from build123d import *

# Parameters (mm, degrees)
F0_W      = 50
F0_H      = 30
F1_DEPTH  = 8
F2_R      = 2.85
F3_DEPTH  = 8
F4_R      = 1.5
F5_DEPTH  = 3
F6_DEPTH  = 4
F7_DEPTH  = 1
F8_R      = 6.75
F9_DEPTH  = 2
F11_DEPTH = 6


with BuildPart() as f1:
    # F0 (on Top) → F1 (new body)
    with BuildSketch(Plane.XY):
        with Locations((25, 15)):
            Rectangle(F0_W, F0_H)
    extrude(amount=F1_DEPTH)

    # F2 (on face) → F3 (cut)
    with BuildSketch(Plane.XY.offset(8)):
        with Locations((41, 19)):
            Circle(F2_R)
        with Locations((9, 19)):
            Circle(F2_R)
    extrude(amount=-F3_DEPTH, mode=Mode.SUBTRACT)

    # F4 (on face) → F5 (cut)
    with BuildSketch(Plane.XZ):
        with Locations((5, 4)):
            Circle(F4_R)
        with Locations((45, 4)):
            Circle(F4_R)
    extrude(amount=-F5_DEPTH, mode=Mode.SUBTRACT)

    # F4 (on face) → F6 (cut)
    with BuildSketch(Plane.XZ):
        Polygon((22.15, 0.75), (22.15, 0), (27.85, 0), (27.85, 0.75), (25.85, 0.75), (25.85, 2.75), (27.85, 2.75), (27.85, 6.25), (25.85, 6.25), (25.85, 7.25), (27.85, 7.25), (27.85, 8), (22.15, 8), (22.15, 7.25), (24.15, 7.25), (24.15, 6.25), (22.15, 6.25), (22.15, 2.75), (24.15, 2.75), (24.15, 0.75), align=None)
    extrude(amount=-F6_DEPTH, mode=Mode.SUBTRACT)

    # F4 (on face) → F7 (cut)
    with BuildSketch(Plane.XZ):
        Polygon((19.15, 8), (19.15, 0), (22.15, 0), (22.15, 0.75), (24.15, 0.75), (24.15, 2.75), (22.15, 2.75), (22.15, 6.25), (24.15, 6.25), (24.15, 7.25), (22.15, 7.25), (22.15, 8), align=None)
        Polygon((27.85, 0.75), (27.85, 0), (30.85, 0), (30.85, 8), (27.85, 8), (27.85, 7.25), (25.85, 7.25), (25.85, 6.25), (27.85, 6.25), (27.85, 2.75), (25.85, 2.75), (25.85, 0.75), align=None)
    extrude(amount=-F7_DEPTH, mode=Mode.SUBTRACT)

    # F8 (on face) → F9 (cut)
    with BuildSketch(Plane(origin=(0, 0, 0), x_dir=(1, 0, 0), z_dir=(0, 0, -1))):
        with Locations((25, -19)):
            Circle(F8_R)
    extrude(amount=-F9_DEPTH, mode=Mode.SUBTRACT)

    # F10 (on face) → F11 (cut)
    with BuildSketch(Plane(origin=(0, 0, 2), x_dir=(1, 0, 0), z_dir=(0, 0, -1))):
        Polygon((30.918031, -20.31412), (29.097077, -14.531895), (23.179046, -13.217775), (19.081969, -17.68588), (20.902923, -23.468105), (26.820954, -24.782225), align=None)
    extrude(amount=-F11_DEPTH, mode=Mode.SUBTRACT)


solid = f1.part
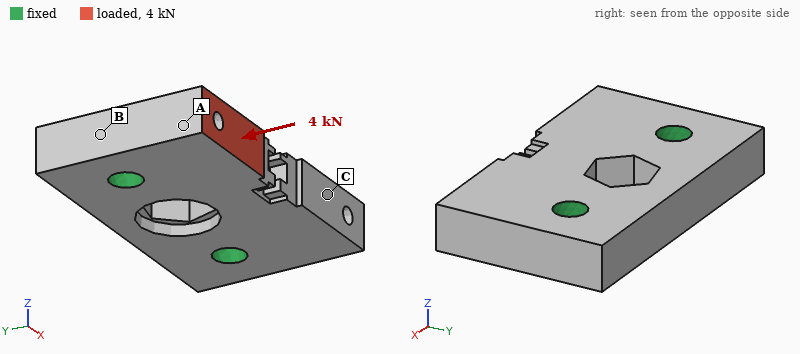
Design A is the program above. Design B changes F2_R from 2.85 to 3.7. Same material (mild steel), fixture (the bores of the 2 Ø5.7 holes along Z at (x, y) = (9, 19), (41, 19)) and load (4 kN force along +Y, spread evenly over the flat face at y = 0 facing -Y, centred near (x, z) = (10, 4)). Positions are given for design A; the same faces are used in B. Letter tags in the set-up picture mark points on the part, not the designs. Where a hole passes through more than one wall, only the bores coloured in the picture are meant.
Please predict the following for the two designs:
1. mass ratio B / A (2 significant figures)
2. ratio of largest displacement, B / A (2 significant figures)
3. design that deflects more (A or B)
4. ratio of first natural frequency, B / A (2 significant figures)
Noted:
0.97
0.91
A
1.1
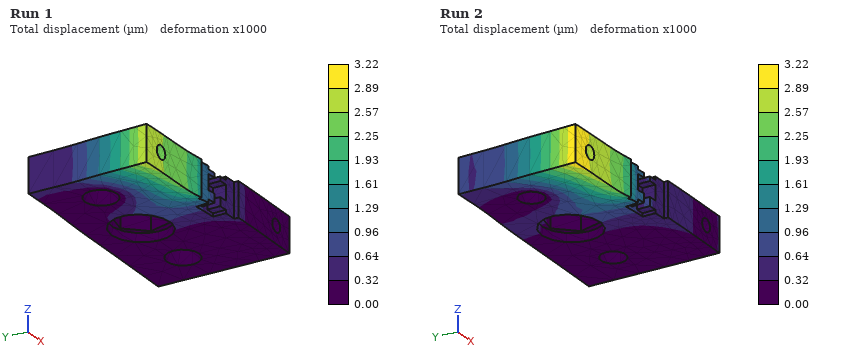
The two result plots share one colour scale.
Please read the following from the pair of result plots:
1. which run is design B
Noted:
Run 1
